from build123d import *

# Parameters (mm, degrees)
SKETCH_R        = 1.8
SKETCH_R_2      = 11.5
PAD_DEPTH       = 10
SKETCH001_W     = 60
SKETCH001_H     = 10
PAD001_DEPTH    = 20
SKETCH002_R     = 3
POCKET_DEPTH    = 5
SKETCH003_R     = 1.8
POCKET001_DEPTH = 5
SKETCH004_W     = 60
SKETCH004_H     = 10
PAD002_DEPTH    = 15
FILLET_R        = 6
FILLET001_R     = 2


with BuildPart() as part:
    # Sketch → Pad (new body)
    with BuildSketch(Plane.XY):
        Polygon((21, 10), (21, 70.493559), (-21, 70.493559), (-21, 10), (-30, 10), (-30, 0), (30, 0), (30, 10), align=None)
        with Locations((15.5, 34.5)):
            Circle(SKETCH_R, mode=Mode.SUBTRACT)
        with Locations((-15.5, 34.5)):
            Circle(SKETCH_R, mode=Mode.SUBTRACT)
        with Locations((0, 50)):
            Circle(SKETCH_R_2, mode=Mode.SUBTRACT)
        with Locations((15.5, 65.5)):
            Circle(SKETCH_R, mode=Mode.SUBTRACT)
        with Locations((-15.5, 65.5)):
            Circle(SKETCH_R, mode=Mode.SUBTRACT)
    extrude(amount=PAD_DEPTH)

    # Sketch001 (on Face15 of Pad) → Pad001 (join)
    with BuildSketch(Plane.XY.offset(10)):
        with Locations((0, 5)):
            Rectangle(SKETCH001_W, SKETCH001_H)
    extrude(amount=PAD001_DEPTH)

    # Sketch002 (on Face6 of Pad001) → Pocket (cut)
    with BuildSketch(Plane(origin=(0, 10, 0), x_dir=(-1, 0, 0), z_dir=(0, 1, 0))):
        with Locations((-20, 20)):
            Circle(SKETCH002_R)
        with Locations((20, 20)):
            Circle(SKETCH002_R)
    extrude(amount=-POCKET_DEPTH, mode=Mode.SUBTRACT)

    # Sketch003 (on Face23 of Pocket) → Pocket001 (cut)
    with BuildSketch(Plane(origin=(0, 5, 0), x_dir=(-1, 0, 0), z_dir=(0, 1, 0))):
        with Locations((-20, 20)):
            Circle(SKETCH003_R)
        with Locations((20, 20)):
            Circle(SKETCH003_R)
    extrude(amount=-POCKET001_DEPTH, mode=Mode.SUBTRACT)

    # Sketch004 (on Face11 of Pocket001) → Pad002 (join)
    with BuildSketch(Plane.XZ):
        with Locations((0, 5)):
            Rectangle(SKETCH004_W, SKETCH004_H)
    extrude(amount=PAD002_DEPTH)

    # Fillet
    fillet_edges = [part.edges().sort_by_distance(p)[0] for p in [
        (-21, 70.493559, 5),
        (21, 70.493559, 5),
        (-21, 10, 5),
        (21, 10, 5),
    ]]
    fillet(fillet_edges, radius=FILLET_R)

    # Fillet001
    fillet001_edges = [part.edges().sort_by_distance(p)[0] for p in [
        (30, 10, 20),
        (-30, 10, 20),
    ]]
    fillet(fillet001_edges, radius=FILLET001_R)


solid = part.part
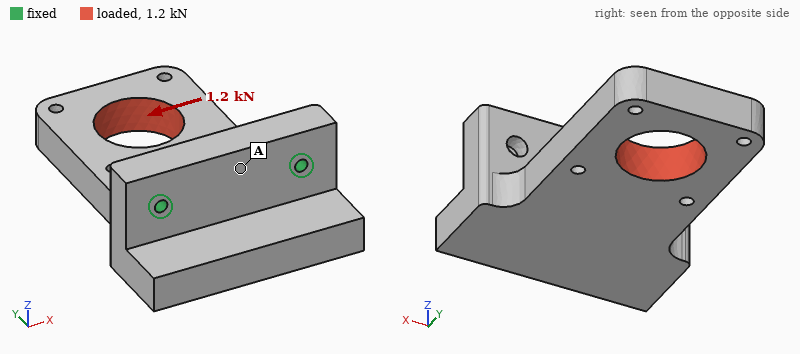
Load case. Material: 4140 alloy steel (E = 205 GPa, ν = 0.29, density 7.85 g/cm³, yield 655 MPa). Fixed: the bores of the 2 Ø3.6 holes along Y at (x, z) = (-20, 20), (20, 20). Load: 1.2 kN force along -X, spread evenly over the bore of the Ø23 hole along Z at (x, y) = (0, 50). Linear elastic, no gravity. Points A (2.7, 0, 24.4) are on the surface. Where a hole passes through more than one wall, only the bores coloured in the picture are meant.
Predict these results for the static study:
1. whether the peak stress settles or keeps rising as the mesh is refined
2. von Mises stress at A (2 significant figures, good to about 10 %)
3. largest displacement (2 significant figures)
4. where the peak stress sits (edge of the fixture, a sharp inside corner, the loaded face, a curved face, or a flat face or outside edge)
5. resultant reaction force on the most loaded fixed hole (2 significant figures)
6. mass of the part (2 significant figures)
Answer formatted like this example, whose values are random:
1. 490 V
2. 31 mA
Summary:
1. keeps rising
2. 10 MPa
3. 24 µm
4. edge of the fixture
5. 1.6 kN
6. 370 g
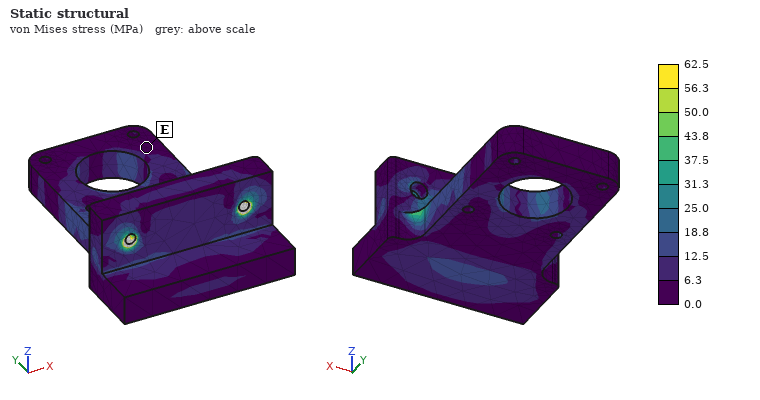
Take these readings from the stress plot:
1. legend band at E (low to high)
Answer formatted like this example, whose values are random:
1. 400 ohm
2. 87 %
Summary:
1. 0.0 to 6.3 MPa
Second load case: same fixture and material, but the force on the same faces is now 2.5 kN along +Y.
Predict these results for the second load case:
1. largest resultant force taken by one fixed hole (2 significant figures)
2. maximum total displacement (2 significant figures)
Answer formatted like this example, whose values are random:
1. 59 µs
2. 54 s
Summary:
1. 1.3 kN
2. 96 µm
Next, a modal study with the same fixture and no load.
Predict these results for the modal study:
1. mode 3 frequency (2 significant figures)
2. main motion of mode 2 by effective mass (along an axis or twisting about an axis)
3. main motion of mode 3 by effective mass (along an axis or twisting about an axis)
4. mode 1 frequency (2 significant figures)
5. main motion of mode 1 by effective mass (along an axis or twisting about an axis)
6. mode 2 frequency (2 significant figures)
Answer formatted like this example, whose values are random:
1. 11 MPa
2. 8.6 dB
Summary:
1. 4600 Hz
2. along X
3. along Y
4. 1200 Hz
5. along Z
6. 3800 Hz
